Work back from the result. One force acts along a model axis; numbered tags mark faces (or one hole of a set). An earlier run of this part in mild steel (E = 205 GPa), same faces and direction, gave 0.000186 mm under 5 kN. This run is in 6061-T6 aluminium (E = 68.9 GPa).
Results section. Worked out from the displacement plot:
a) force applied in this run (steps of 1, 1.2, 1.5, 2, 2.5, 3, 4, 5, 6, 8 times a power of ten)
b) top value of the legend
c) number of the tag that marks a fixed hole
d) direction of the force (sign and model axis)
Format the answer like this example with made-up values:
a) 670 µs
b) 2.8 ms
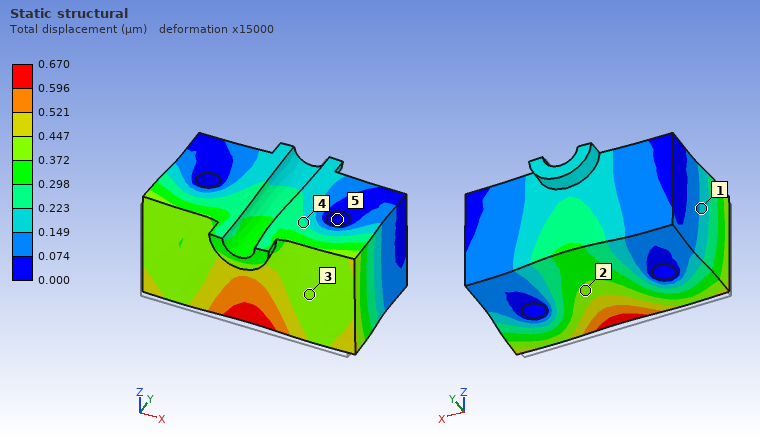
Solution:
a) 6 kN
b) 0.670 µm
c) 5
d) +Y
